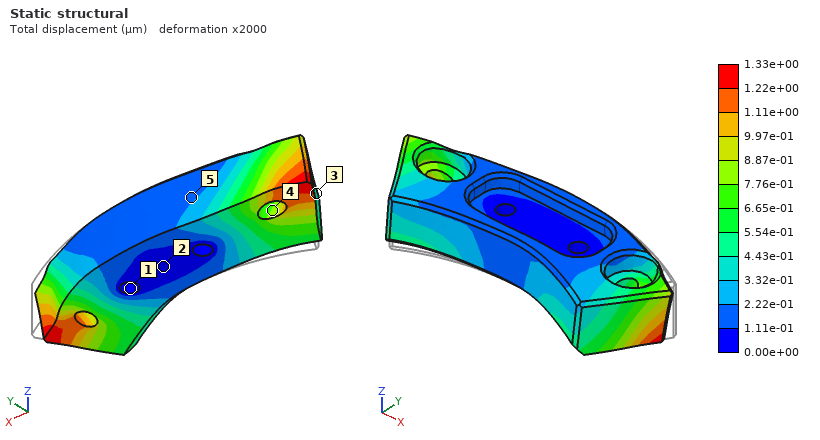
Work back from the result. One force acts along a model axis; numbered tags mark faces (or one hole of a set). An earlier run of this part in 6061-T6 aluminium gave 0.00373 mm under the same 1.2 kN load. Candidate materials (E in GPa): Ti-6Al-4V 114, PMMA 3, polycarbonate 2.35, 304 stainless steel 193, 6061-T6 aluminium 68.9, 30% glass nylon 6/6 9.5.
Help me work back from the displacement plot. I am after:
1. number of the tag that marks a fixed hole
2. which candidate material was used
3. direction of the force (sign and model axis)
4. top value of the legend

1
304 stainless steel
-X
1.33e+00 µm
